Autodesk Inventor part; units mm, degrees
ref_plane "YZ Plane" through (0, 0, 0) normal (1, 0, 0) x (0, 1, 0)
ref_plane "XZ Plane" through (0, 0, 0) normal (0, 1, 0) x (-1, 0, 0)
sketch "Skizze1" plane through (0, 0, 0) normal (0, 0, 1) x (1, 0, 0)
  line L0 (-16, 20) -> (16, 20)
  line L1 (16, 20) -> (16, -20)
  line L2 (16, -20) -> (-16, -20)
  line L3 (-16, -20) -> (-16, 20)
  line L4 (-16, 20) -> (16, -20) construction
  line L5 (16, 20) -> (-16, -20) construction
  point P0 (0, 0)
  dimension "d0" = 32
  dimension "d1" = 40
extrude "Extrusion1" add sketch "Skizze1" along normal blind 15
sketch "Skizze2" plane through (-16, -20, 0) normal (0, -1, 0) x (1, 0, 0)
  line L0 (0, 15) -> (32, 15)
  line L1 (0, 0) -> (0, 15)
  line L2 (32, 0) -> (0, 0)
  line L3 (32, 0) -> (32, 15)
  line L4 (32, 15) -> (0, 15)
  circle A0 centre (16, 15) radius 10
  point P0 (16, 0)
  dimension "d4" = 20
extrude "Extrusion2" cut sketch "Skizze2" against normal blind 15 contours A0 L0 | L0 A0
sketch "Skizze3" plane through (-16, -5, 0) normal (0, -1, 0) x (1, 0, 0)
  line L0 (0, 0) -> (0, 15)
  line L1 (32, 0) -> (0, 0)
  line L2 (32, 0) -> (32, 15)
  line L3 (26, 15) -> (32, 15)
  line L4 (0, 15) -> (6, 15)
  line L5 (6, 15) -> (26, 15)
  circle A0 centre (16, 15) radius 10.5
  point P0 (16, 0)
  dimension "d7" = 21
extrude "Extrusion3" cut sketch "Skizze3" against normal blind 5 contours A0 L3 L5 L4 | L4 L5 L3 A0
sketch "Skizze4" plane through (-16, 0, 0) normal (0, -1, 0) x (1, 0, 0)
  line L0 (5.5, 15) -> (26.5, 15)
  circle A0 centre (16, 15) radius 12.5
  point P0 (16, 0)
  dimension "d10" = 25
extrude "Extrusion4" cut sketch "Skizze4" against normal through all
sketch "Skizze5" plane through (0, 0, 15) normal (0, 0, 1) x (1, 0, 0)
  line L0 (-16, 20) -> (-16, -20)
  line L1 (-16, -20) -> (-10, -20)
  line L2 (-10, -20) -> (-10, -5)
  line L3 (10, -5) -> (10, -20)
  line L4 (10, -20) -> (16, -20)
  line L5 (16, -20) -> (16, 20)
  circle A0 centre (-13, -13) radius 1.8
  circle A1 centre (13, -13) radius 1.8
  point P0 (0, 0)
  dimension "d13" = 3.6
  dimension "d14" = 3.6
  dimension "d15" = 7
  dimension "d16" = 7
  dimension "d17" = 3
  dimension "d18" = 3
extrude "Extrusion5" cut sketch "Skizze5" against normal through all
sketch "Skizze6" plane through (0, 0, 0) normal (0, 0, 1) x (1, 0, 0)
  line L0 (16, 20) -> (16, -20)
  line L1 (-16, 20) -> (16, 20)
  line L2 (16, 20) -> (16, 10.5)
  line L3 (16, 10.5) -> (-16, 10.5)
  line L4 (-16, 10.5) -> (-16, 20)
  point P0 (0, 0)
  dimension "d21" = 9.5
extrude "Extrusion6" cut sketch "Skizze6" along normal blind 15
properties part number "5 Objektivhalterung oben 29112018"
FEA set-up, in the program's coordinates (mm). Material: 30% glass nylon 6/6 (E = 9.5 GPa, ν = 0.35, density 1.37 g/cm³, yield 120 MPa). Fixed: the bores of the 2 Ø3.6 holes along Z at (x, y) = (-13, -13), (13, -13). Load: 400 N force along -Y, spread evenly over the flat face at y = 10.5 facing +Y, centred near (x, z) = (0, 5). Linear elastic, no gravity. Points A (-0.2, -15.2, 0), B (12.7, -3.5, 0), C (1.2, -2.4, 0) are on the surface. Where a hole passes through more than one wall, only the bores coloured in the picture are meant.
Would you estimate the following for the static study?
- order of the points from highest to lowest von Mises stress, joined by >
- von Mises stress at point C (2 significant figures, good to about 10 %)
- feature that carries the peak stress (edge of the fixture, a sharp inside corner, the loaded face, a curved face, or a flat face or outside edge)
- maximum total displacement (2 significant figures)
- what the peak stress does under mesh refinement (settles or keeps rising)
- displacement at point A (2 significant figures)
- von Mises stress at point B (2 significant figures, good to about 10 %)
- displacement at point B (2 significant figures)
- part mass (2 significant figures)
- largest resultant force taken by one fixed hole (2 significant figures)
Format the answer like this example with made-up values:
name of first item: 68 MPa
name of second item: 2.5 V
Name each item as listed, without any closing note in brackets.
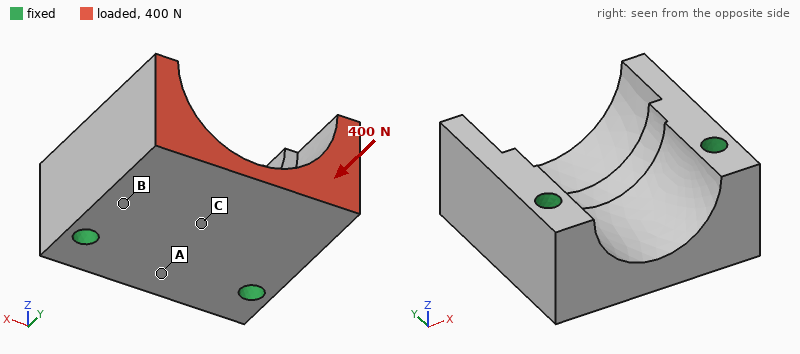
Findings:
order of the points from highest to lowest von Mises stress, joined by >: B > C > A
von Mises stress at point C: 1.2 MPa
feature that carries the peak stress: edge of the fixture
maximum total displacement: 6.3 µm
what the peak stress does under mesh refinement: keeps rising
displacement at point A: 2.1 µm
von Mises stress at point B: 2.1 MPa
displacement at point B: 2.6 µm
part mass: 12 g
largest resultant force taken by one fixed hole: 200 N
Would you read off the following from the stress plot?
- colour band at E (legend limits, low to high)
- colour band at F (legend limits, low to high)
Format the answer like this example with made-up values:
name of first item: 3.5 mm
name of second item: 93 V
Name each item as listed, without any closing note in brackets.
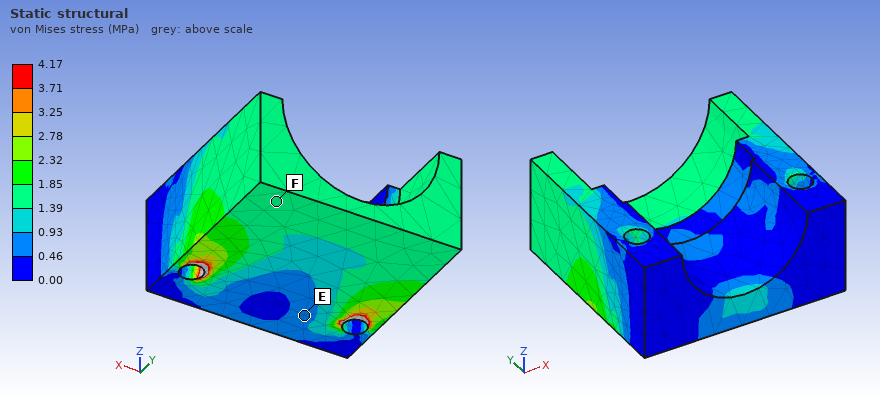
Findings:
colour band at E: 0.46 to 0.93 MPa
colour band at F: 1.39 to 1.85 MPa
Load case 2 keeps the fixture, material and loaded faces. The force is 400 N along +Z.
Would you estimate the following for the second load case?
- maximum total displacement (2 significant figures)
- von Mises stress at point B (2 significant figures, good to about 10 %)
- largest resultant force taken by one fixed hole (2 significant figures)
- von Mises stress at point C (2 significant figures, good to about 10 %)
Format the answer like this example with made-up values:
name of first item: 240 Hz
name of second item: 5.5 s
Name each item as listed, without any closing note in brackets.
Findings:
maximum total displacement: 72 µm
von Mises stress at point B: 9.3 MPa
largest resultant force taken by one fixed hole: 200 N
von Mises stress at point C: 4.6 MPa
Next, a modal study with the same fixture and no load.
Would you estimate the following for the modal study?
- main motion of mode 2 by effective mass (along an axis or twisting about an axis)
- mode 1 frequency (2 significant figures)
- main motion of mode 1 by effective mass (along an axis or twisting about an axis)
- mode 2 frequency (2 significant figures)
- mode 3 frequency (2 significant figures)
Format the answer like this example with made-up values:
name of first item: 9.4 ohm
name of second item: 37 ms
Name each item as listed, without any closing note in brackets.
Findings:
main motion of mode 2 by effective mass: along X
mode 1 frequency: 9100 Hz
main motion of mode 1 by effective mass: along Z
mode 2 frequency: 9600 Hz
mode 3 frequency: 12 kHz
